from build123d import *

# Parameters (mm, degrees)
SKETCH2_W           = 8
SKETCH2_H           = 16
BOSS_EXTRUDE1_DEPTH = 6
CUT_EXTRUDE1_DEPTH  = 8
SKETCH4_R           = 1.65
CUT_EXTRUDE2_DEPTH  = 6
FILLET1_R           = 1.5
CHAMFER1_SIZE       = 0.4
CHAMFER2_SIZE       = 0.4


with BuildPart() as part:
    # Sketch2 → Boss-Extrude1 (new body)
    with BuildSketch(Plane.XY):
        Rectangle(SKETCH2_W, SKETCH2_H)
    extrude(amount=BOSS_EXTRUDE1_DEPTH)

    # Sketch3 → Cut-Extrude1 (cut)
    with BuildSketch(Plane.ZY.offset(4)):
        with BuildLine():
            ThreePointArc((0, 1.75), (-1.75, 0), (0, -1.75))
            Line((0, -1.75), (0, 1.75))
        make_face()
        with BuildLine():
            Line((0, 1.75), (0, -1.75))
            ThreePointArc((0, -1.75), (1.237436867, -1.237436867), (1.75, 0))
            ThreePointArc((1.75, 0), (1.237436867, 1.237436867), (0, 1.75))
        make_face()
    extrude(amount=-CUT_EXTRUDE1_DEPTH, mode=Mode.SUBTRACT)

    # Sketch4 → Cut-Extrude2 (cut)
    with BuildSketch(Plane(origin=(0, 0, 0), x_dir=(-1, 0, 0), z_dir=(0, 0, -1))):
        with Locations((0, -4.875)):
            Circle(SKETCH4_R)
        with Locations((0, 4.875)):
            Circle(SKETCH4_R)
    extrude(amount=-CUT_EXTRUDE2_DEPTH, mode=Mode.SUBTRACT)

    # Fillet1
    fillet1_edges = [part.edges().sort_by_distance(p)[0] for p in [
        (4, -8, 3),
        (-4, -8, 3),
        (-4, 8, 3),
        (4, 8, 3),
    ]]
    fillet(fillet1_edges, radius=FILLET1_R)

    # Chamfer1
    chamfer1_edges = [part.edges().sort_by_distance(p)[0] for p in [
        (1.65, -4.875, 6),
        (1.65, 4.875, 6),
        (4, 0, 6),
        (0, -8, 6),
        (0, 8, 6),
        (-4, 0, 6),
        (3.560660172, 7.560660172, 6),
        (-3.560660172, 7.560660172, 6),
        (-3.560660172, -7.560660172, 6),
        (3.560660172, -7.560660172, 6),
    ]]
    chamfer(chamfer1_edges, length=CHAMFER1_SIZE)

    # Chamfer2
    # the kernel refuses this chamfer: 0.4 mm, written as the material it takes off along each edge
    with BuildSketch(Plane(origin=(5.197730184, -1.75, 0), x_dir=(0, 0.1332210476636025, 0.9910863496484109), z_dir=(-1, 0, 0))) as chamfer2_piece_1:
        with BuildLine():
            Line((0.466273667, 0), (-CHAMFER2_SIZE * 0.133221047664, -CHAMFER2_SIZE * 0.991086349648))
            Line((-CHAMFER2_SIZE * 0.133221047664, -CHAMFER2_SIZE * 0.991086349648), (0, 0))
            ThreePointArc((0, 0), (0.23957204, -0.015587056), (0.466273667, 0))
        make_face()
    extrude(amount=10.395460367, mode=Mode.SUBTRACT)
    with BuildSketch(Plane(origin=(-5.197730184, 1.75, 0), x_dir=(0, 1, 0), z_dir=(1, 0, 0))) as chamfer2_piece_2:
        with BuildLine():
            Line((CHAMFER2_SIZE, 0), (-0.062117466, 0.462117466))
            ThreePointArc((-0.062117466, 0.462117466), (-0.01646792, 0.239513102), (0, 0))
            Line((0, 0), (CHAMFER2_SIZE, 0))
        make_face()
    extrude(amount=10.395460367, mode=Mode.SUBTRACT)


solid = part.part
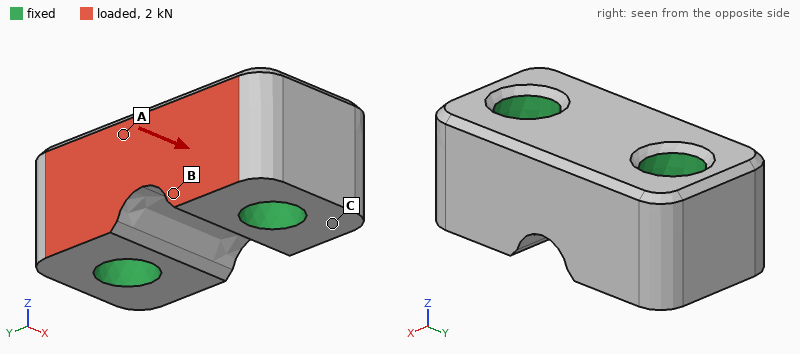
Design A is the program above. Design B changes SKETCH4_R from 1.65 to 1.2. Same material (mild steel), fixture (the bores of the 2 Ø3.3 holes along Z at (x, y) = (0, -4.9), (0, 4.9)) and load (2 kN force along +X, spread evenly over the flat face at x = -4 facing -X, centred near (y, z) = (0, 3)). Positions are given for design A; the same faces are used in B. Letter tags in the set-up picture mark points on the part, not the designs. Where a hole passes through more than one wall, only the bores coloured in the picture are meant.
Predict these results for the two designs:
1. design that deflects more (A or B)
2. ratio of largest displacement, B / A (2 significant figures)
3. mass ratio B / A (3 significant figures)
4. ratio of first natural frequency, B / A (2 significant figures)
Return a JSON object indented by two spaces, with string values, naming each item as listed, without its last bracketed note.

{
  "design that deflects more": "B",
  "ratio of largest displacement, B / A": "1.2",
  "mass ratio B / A": "1.08",
  "ratio of first natural frequency, B / A": "0.82"
}
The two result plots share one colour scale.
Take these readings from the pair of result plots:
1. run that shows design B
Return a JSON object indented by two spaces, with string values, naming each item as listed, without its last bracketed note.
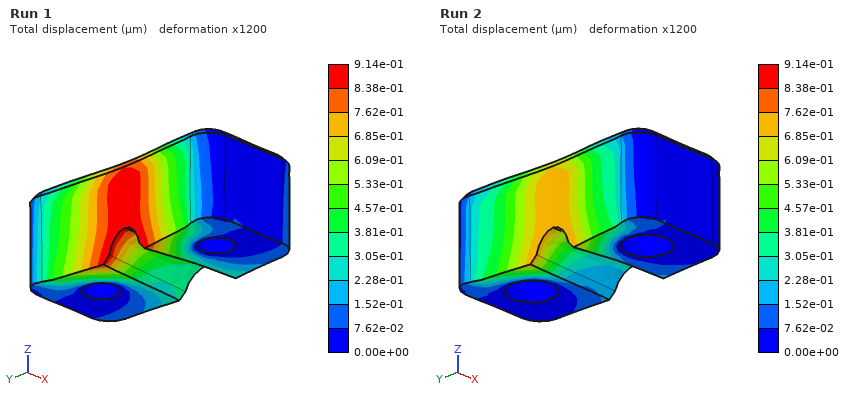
{
  "run that shows design B": "Run 1"
}
